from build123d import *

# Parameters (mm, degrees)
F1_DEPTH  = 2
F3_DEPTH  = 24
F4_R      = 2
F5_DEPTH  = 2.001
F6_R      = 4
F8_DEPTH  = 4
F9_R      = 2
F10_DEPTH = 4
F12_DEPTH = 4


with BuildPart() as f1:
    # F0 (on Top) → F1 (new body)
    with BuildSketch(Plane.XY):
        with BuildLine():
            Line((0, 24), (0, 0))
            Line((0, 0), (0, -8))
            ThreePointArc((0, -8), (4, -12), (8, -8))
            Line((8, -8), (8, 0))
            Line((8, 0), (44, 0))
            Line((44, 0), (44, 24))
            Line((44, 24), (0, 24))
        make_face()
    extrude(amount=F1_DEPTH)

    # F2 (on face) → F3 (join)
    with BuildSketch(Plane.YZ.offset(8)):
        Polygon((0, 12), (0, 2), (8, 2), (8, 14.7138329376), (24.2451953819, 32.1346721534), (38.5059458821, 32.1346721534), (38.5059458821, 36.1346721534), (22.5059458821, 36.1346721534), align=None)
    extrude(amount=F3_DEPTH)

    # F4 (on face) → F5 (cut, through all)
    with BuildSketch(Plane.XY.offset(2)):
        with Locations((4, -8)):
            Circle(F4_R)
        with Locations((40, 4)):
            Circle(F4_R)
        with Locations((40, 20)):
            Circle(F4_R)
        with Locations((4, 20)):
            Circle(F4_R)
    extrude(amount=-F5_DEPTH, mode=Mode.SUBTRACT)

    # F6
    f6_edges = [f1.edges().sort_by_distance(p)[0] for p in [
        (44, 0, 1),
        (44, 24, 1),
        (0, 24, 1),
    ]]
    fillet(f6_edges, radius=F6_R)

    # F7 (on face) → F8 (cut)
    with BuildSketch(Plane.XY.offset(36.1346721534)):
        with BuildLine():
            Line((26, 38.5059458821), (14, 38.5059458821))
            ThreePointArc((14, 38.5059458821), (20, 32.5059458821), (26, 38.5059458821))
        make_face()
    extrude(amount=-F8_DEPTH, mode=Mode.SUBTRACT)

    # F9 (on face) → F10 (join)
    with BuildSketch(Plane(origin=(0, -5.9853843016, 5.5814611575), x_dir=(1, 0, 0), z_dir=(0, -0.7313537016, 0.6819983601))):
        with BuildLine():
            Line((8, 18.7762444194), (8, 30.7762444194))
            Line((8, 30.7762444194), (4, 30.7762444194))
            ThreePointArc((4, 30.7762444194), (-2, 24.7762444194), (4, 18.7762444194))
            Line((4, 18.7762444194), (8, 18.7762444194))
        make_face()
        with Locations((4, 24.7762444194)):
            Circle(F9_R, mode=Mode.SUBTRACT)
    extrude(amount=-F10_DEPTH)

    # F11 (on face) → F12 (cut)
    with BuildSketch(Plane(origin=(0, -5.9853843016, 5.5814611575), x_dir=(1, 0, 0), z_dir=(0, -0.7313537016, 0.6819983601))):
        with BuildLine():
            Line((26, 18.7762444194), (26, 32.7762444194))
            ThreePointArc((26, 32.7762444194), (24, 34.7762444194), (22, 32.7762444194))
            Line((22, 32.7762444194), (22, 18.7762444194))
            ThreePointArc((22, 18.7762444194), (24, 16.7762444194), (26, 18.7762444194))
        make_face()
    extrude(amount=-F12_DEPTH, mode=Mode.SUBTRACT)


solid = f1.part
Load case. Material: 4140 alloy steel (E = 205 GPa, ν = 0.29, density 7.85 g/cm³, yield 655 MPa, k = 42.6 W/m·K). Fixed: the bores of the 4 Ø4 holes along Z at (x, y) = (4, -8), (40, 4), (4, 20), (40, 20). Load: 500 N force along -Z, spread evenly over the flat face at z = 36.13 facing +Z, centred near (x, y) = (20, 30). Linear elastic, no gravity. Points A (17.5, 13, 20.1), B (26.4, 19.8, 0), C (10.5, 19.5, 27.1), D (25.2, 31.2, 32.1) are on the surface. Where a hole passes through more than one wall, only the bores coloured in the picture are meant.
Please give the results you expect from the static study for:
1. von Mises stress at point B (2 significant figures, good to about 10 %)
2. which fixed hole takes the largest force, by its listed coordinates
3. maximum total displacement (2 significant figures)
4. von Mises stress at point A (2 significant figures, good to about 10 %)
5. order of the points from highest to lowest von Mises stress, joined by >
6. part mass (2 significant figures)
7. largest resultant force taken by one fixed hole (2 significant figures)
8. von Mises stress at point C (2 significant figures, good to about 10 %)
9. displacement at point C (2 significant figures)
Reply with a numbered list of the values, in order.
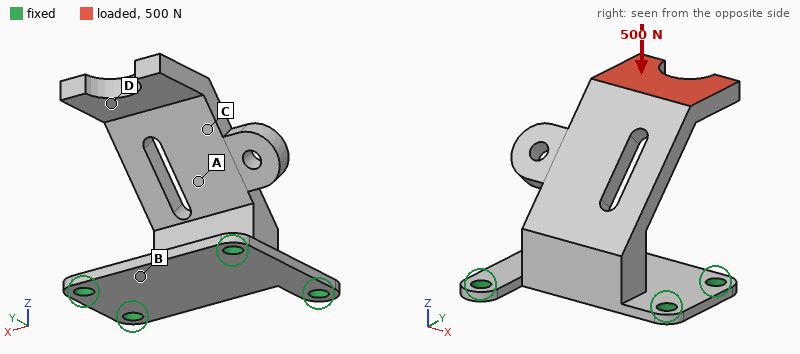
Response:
1. 62 MPa
2. (4, 20)
3. 0.56 mm
4. 160 MPa
5. A > C > B > D
6. 66 g
7. 510 N
8. 110 MPa
9. 0.26 mm
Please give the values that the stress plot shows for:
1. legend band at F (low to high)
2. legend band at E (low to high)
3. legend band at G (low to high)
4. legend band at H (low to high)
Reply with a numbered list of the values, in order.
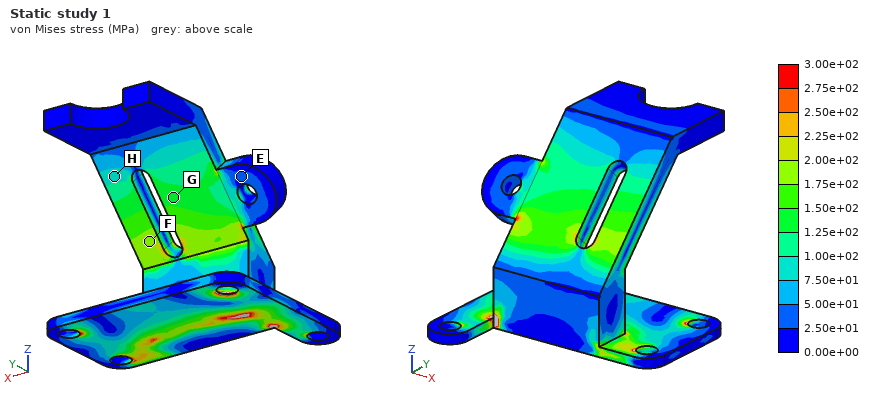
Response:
1. 1.75e+02 to 2.00e+02 MPa
2. 2.50e+01 to 5.00e+01 MPa
3. 1.25e+02 to 1.50e+02 MPa
4. 7.50e+01 to 1.00e+02 MPa
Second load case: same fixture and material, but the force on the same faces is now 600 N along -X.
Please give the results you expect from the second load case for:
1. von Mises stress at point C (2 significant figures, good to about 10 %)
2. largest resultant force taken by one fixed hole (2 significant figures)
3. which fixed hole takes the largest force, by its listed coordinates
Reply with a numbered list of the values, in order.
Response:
1. 44 MPa
2. 790 N
3. (40, 4)
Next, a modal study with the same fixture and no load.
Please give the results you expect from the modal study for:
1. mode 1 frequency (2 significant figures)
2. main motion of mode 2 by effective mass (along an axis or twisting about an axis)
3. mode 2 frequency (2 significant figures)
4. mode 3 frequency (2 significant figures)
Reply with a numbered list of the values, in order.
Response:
1. 1100 Hz
2. along X
3. 2600 Hz
4. 4100 Hz
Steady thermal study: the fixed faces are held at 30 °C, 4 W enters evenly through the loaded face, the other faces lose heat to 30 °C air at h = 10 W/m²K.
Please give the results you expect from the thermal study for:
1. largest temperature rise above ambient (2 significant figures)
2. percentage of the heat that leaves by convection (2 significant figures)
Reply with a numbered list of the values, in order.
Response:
1. 48 K
2. 24 %
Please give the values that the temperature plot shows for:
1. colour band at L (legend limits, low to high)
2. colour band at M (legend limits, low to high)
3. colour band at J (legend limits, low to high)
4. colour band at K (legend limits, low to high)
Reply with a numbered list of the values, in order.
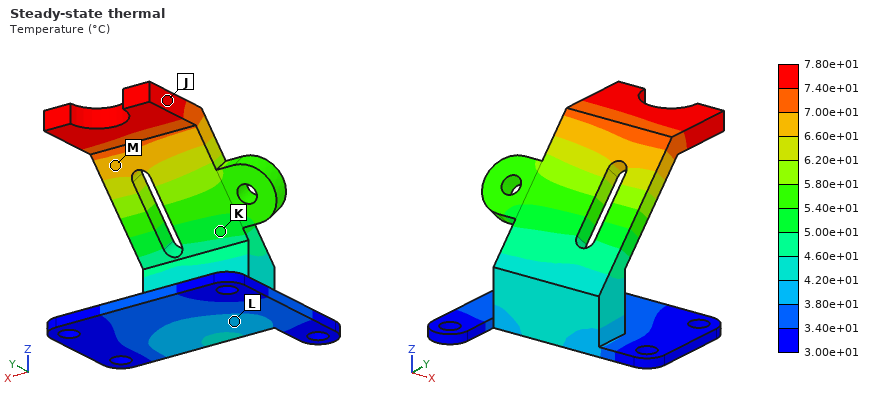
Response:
1. 3.80e+01 to 4.20e+01 °C
2. 6.60e+01 to 7.00e+01 °C
3. 7.40e+01 to 7.80e+01 °C
4. 5.00e+01 to 5.40e+01 °C
